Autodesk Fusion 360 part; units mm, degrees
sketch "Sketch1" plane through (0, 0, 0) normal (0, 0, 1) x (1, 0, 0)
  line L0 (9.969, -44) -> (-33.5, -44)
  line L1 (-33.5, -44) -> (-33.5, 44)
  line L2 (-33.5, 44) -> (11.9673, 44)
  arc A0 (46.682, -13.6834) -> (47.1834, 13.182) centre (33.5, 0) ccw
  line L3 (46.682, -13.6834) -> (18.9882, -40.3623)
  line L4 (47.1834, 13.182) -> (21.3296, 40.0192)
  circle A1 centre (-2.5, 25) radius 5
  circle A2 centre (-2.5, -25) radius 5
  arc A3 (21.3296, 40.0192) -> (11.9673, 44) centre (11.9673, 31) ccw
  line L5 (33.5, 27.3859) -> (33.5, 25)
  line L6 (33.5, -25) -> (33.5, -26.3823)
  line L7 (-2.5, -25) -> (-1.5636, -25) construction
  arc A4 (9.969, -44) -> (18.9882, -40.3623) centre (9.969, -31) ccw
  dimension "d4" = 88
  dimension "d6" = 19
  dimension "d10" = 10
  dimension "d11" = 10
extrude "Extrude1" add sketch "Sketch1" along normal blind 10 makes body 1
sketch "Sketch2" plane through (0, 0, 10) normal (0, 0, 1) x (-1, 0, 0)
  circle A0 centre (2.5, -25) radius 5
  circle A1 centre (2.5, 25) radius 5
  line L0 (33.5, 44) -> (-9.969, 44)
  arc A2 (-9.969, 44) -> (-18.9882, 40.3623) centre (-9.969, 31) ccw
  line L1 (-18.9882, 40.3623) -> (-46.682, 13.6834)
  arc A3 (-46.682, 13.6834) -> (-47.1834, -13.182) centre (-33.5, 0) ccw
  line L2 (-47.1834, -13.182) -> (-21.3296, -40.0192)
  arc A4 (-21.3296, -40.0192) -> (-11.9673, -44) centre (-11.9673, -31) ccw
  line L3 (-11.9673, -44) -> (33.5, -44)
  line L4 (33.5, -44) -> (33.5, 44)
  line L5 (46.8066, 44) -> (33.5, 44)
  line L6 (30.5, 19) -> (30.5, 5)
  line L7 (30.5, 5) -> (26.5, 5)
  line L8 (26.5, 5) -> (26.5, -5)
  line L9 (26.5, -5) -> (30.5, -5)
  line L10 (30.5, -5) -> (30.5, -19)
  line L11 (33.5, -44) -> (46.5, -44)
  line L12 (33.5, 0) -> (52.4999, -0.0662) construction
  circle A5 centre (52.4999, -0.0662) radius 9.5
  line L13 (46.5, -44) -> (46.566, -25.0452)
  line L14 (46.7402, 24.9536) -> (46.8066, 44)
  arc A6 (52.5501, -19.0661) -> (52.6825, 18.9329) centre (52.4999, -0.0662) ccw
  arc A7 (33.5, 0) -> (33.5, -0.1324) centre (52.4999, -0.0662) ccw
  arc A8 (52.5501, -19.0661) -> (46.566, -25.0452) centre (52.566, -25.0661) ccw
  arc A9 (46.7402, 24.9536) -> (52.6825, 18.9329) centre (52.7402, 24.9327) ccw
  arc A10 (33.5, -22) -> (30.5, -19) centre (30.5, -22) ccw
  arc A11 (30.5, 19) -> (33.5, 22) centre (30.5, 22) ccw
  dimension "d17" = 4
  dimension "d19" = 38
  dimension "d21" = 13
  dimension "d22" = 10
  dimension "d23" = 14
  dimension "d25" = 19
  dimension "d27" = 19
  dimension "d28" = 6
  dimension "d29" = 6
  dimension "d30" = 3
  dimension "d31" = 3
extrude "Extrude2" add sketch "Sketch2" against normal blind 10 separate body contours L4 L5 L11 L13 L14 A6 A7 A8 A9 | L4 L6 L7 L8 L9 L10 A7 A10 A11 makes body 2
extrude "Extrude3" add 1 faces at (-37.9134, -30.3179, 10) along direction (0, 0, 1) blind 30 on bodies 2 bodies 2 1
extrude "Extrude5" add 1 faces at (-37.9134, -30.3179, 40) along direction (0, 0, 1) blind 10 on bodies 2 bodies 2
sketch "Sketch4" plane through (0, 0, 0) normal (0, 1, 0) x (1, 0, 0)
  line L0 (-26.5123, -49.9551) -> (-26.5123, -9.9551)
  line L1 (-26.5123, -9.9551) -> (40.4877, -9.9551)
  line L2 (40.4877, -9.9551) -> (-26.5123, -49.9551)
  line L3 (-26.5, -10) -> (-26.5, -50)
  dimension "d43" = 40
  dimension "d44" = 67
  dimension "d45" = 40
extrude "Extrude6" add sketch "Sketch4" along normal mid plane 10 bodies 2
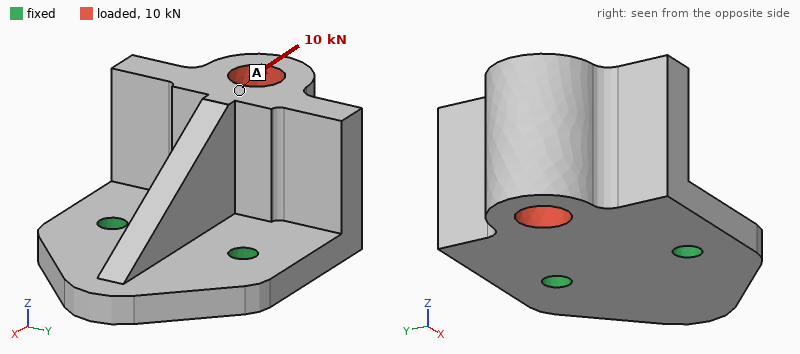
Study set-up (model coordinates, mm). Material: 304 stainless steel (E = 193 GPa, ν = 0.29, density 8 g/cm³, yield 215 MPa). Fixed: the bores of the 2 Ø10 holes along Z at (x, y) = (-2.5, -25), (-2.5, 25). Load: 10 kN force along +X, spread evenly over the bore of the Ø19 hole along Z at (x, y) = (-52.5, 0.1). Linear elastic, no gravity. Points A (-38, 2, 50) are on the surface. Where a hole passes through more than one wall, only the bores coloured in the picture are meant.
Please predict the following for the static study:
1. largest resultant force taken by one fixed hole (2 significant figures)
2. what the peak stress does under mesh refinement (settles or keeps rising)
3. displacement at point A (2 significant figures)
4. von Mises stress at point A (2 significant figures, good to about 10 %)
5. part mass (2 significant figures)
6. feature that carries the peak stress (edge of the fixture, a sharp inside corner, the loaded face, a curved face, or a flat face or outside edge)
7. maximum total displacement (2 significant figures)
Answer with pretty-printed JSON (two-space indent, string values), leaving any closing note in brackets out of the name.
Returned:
{
  "largest resultant force taken by one fixed hole": "5.0 kN",
  "what the peak stress does under mesh refinement": "keeps rising",
  "displacement at point A": "67 µm",
  "von Mises stress at point A": "20 MPa",
  "part mass": "1.3 kg",
  "feature that carries the peak stress": "edge of the fixture",
  "maximum total displacement": "98 µm"
}
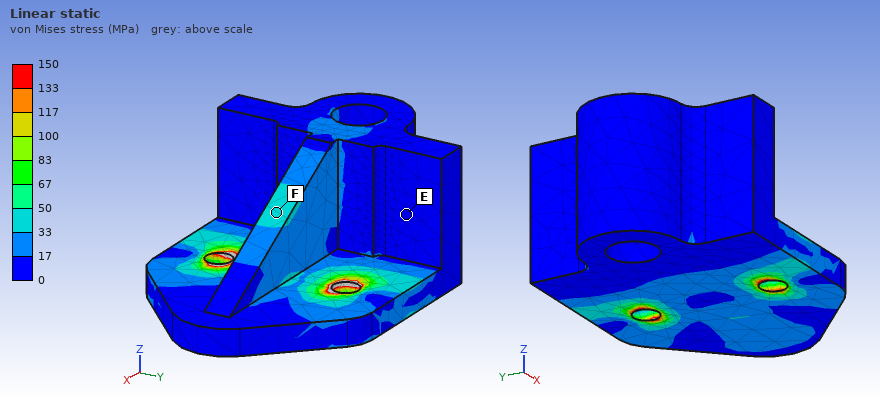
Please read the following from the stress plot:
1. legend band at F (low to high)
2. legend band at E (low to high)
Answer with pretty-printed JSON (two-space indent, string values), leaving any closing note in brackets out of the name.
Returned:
{
  "legend band at F": "33 to 50 MPa",
  "legend band at E": "0 to 17 MPa"
}
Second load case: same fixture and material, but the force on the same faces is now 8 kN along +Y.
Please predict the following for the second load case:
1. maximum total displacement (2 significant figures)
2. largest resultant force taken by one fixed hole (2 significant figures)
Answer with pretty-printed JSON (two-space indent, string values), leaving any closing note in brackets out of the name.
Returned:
{
  "maximum total displacement": "40 µm",
  "largest resultant force taken by one fixed hole": "8.7 kN"
}
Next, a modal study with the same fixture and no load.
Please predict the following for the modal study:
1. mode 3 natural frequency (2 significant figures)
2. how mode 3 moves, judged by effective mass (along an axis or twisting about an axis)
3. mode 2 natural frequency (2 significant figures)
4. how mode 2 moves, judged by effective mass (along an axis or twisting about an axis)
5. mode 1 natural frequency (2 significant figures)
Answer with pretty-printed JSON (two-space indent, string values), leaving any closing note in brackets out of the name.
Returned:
{
  "mode 3 natural frequency": "5300 Hz",
  "how mode 3 moves, judged by effective mass": "along Z",
  "mode 2 natural frequency": "2800 Hz",
  "how mode 2 moves, judged by effective mass": "along Y",
  "mode 1 natural frequency": "1500 Hz"
}
